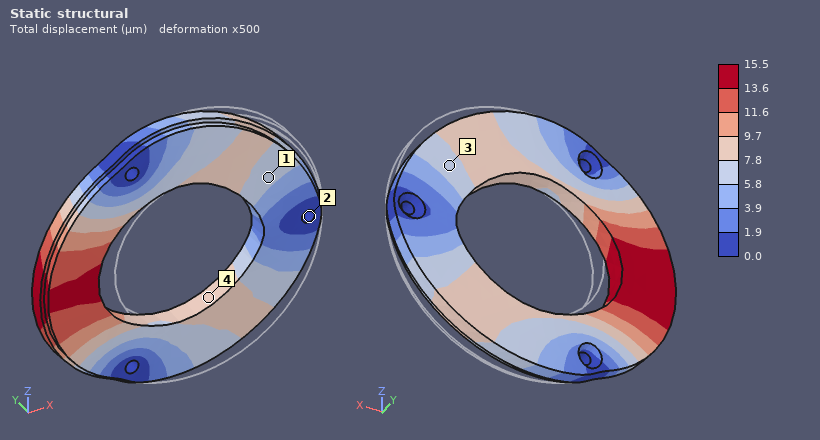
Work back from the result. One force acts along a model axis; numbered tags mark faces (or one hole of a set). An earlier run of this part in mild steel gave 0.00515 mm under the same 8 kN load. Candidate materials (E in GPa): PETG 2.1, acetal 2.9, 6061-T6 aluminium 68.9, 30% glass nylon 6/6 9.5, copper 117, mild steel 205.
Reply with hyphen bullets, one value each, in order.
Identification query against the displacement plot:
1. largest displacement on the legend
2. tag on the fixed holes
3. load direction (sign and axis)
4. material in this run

- 15.5 µm
- 2
- -X
- 6061-T6 aluminium
